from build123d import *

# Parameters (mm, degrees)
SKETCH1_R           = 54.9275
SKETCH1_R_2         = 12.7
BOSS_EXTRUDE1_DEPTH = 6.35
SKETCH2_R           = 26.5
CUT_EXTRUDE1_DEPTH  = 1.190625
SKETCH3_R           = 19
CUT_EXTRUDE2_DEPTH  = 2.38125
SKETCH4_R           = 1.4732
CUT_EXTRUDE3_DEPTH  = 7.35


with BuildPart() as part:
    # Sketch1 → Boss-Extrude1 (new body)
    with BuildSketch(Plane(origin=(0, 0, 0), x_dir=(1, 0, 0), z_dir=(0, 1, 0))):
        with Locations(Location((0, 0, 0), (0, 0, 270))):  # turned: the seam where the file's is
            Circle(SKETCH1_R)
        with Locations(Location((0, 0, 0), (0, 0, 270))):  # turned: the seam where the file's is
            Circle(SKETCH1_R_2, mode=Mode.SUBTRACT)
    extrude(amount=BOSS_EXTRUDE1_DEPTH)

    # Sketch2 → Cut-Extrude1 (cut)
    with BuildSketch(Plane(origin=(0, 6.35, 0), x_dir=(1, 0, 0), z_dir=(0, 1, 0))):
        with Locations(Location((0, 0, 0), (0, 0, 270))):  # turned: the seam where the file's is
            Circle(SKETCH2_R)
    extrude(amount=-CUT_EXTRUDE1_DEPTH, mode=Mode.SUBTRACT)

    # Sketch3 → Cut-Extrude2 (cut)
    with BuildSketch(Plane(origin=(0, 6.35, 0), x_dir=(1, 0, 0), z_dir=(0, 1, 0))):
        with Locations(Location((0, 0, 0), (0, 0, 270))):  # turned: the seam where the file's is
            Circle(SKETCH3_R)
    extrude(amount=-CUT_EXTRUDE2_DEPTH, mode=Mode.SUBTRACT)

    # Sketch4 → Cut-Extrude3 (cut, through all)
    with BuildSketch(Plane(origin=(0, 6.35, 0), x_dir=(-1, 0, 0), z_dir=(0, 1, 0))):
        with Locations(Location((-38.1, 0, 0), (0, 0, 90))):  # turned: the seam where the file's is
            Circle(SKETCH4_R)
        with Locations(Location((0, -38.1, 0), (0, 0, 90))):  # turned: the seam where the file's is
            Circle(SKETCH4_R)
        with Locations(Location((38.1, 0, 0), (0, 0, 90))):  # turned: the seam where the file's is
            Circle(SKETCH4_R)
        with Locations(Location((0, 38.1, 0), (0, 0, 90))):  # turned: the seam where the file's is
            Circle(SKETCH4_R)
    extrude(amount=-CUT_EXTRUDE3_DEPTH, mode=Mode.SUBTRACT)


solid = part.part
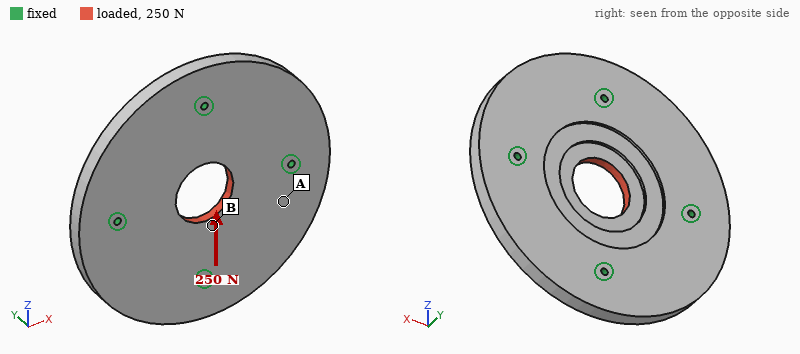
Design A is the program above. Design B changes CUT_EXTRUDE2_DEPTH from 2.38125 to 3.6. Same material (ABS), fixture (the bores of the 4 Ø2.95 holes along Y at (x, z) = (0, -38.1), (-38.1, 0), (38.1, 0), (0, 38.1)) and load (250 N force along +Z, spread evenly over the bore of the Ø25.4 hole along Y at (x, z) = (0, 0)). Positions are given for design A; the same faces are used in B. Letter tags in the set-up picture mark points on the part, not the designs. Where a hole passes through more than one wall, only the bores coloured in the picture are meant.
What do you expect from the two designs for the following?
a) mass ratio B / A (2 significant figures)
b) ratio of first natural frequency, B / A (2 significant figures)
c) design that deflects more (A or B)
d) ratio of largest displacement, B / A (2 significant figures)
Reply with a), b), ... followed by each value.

a) 0.99
b) 1.00
c) B
d) 1.6
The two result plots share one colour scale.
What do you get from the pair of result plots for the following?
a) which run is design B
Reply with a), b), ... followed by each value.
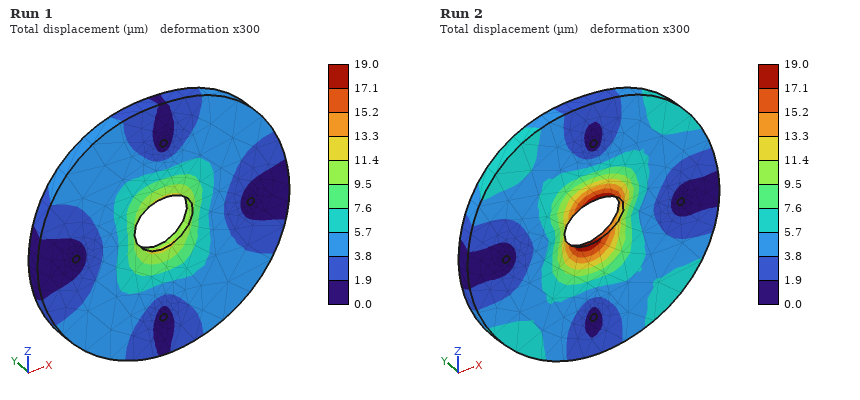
a) Run 2
